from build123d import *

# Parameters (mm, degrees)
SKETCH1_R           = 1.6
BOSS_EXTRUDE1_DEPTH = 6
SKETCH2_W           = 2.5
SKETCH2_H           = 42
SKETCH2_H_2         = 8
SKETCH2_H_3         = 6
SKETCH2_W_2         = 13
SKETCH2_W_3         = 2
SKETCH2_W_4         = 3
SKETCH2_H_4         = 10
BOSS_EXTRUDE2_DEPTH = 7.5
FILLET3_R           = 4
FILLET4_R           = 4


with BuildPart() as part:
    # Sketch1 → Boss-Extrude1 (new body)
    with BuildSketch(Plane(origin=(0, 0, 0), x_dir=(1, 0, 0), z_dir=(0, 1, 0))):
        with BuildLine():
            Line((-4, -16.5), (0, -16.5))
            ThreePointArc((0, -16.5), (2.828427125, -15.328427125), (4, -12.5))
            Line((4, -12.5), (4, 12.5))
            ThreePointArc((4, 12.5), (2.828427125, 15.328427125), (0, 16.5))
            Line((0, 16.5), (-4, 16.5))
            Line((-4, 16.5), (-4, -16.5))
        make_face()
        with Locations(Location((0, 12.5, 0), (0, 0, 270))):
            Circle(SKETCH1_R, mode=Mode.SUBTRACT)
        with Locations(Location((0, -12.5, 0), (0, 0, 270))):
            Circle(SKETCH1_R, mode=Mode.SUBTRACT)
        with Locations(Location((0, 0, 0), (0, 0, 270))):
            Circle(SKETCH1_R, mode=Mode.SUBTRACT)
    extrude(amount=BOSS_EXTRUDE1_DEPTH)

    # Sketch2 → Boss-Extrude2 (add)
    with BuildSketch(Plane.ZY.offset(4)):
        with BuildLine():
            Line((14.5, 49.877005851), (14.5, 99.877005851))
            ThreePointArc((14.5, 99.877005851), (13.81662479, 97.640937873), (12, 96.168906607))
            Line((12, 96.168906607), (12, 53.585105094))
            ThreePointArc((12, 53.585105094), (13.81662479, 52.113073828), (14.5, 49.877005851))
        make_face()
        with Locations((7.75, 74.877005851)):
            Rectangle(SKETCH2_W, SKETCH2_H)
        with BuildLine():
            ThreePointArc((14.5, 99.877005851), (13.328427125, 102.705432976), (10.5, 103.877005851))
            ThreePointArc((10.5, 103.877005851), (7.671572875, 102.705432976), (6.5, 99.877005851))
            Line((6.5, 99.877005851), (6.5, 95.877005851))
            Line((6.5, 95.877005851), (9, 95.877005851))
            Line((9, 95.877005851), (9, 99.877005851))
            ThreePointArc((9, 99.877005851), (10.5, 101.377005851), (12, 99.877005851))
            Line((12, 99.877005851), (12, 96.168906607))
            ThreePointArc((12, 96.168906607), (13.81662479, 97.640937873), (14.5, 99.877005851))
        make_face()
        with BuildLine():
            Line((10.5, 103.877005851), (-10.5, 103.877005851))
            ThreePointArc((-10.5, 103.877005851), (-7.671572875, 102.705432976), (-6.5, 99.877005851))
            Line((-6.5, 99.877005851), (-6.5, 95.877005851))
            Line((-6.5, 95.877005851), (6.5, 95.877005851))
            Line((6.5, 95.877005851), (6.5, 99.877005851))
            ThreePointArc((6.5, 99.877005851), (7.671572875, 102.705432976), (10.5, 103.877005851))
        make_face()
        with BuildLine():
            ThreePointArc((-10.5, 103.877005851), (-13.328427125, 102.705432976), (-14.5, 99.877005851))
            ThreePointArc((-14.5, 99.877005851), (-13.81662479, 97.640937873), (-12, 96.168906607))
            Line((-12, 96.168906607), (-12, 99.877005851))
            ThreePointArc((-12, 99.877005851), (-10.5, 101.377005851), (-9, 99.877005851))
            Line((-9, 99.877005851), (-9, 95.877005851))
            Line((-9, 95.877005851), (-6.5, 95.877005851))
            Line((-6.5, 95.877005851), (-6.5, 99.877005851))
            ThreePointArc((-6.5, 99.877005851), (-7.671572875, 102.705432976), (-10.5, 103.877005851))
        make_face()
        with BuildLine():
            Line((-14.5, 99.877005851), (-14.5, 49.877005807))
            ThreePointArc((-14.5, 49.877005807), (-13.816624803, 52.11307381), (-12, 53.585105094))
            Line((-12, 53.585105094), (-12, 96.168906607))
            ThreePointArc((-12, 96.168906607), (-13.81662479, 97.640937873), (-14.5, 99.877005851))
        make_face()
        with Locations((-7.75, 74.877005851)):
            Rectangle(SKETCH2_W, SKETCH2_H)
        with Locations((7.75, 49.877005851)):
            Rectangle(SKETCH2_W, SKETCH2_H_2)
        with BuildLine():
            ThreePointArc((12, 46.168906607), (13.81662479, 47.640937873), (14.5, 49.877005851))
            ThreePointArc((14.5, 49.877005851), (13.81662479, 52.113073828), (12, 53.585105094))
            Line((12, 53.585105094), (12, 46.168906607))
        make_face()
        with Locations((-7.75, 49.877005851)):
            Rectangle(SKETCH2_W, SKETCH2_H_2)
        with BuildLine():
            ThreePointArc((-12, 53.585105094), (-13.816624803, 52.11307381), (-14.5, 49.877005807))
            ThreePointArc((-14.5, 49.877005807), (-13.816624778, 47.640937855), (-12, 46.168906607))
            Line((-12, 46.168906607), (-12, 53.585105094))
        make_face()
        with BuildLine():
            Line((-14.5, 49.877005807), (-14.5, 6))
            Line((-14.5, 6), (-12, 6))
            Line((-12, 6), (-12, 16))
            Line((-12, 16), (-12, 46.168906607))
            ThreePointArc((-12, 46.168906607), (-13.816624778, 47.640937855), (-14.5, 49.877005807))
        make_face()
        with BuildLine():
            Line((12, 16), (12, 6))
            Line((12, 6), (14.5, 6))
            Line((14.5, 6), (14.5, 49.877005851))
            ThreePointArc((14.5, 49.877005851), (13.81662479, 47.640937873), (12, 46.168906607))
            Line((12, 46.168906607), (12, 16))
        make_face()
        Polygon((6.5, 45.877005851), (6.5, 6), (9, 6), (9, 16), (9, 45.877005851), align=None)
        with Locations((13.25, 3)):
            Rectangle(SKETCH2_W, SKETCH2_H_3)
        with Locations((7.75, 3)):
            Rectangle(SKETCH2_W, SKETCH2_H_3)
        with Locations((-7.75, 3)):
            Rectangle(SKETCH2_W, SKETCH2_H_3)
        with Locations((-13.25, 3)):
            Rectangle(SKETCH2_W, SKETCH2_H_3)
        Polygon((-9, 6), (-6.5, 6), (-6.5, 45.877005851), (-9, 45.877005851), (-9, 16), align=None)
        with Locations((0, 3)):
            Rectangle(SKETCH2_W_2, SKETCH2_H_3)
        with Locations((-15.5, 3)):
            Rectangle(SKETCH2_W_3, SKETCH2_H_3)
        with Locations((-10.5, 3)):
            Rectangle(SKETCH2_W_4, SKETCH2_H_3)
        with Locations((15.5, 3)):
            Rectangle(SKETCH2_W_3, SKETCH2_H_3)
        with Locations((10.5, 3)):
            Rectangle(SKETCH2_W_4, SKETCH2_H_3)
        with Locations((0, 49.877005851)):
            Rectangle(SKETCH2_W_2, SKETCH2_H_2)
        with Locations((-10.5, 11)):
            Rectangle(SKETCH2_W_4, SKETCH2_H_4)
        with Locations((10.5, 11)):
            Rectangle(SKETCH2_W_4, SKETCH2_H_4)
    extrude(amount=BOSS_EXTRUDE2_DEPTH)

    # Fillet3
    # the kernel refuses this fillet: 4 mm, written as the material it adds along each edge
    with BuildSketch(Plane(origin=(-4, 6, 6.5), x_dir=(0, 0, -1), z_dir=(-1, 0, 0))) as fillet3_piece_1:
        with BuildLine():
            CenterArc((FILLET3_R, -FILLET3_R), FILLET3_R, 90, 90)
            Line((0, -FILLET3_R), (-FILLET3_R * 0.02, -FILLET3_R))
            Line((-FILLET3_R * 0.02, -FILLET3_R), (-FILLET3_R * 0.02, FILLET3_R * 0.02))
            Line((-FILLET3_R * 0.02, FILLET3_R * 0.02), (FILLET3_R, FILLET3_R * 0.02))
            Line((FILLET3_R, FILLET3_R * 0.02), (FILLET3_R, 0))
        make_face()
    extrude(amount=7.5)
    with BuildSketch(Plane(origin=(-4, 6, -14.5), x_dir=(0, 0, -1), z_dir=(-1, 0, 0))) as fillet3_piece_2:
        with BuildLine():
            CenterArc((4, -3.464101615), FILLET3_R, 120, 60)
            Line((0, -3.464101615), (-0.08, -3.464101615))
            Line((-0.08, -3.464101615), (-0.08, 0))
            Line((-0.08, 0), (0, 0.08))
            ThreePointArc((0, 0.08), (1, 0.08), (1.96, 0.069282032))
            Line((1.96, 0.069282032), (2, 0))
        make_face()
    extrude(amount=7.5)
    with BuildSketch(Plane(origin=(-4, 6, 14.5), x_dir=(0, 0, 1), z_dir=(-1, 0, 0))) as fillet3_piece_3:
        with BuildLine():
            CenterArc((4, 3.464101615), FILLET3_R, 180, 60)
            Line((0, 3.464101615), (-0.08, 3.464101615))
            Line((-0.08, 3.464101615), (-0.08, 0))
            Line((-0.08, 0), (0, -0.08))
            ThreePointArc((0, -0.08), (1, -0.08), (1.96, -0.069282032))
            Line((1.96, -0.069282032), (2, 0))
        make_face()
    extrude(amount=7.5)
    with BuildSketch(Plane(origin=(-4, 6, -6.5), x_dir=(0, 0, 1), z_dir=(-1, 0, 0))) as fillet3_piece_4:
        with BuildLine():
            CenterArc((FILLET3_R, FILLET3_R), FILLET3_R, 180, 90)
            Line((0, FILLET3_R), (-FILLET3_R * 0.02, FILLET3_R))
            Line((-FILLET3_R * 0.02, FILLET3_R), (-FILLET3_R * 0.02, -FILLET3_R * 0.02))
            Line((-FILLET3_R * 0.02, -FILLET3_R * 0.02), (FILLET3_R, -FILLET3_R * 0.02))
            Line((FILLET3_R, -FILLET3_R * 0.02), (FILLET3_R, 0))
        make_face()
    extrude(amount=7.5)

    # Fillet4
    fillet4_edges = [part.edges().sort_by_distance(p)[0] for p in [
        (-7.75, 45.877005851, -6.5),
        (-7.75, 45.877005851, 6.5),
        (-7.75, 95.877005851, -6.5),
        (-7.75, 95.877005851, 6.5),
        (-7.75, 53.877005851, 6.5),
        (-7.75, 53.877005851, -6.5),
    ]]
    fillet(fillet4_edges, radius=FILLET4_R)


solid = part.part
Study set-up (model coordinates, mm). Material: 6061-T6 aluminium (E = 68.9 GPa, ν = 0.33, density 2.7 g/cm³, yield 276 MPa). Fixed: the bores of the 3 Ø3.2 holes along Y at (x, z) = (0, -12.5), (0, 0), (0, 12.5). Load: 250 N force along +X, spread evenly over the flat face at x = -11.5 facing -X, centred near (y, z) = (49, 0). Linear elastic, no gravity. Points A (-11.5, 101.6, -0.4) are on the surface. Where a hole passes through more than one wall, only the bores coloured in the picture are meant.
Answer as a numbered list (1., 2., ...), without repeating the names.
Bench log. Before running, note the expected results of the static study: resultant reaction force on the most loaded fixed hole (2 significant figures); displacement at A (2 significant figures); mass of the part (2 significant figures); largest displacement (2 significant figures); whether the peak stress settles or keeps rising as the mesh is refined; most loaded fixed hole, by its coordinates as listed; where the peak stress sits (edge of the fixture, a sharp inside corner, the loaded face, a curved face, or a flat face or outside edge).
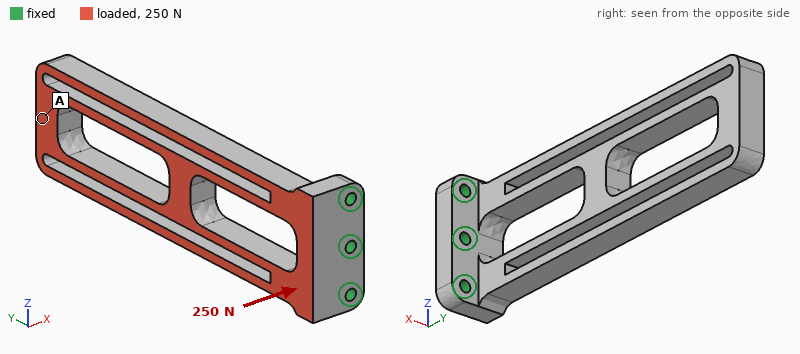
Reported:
1. 150 N
2. 1.2 mm
3. 34 g
4. 1.2 mm
5. keeps rising
6. (0, 0)
7. edge of the fixture
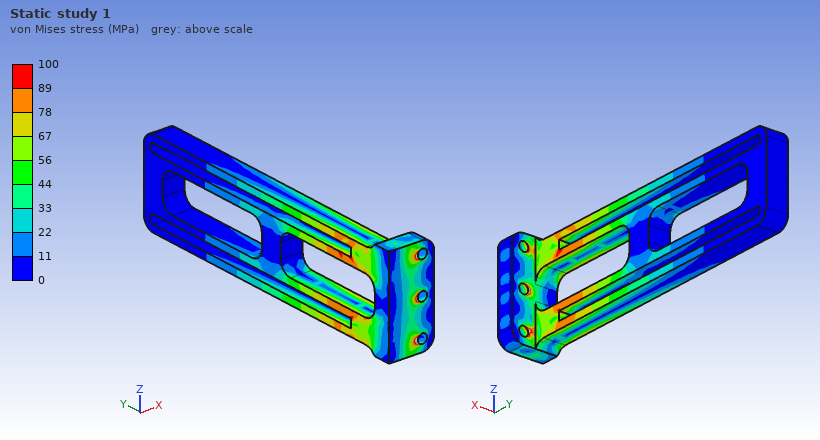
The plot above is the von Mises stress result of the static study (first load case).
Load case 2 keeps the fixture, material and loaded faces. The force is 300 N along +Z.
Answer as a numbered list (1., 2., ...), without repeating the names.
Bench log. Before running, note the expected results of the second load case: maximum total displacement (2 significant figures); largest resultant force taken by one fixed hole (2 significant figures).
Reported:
1. 0.71 mm
2. 520 N
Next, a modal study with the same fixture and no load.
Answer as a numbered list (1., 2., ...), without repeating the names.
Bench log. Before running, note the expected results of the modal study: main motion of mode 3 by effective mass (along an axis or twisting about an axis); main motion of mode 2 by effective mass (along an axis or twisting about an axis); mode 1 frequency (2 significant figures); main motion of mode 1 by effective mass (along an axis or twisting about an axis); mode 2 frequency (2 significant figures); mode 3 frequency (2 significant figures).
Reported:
1. twisting about Y
2. along Z
3. 510 Hz
4. along X
5. 670 Hz
6. 1600 Hz
